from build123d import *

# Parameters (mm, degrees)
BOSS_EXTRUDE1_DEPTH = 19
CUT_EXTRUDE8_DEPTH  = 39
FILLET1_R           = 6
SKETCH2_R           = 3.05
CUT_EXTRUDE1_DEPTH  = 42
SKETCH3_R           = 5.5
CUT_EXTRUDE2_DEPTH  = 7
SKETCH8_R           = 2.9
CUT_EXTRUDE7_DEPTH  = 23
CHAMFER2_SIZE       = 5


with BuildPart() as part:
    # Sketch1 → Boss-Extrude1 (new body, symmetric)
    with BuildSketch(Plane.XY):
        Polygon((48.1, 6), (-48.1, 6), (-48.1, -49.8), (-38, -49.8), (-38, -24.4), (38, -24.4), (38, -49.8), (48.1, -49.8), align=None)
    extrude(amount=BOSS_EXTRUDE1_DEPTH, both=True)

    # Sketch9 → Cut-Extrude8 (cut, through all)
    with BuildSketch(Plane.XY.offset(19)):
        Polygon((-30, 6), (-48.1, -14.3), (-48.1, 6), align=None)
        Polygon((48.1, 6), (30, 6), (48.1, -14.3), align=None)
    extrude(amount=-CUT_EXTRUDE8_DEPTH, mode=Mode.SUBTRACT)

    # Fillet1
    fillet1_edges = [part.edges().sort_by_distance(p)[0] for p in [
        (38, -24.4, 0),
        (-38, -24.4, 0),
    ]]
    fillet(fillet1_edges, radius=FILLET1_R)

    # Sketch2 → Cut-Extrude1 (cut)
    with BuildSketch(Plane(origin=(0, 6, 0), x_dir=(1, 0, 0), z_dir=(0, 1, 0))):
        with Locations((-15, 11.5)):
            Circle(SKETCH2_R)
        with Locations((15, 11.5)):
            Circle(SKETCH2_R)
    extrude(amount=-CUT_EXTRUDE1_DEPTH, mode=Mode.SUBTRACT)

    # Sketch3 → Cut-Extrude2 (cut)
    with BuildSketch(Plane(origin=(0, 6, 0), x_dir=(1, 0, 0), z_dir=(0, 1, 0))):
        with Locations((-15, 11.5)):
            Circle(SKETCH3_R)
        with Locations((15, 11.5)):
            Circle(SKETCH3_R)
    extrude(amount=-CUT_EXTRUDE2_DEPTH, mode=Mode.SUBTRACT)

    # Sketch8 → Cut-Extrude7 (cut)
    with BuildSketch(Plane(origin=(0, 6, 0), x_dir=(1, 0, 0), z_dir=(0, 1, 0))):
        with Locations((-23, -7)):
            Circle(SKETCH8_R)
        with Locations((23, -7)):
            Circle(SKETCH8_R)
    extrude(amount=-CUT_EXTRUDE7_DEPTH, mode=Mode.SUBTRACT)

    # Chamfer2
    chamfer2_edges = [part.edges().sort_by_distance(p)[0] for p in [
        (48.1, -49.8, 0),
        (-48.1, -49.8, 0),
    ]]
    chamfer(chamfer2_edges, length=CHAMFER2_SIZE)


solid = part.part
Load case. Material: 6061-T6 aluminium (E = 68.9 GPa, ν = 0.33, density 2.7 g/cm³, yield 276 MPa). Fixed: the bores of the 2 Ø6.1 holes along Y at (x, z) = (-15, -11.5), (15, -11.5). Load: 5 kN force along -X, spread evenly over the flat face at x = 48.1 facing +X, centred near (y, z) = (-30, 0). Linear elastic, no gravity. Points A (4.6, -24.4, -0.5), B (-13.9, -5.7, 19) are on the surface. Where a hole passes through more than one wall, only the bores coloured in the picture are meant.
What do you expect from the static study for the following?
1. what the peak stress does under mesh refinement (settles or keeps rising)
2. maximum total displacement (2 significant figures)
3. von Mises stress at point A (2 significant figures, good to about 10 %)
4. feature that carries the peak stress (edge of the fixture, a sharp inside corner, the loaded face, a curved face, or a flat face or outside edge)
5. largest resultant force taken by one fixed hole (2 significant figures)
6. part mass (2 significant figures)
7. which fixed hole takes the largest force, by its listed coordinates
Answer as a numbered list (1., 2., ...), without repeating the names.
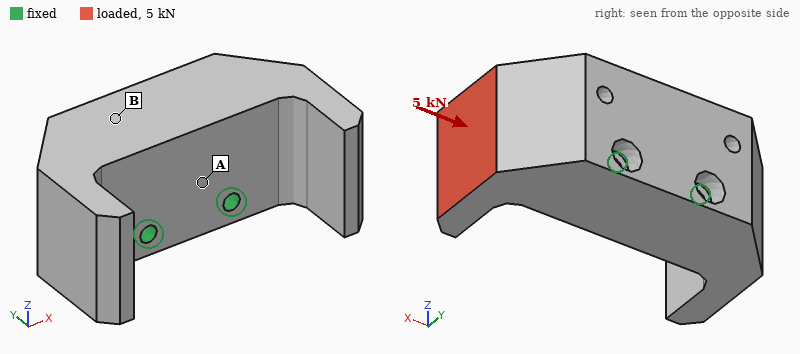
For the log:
1. keeps rising
2. 72 µm
3. 13 MPa
4. edge of the fixture
5. 4.3 kN
6. 300 g
7. (15, -11.5)
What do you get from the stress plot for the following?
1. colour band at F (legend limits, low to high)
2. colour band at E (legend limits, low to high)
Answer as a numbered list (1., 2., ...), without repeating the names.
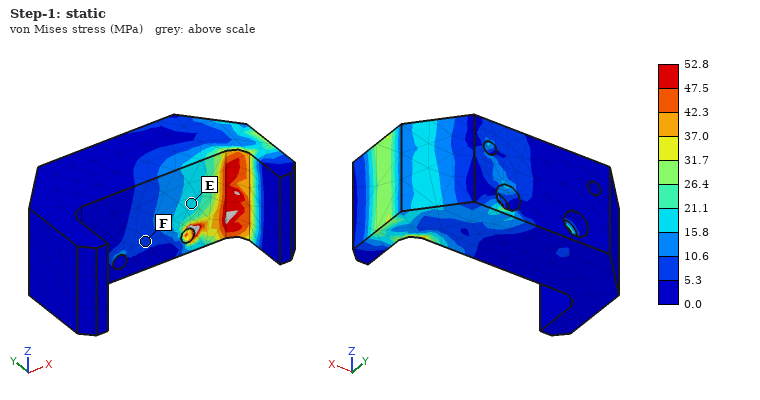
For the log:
1. 5.3 to 10.6 MPa
2. 15.8 to 21.1 MPa
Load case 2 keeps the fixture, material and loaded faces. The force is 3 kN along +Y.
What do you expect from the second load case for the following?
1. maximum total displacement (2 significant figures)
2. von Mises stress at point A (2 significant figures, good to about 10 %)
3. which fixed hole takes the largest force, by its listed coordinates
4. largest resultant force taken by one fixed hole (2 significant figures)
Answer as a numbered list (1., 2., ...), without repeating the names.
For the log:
1. 46 µm
2. 9.7 MPa
3. (15, -11.5)
4. 4.0 kN
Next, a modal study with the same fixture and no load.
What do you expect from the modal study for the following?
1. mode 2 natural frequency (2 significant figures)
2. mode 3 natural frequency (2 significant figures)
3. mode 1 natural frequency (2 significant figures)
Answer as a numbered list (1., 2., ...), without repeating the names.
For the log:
1. 6900 Hz
2. 7100 Hz
3. 6700 Hz
